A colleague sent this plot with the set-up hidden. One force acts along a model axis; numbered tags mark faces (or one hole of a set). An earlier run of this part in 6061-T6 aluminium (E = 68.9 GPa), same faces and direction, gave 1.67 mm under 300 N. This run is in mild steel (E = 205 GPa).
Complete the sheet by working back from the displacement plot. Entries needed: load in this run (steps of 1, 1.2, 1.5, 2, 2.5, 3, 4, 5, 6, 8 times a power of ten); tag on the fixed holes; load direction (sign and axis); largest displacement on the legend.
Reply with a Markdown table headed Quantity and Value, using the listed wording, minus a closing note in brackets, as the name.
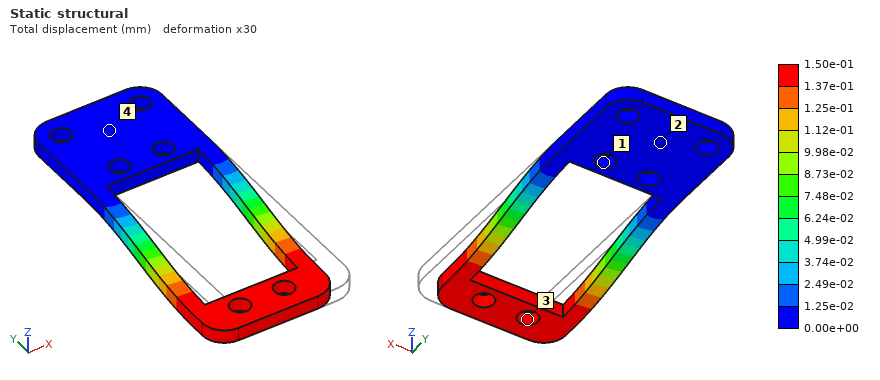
| Quantity | Value |
|---|---|
| load in this run | 80 N |
| tag on the fixed holes | 1 |
| load direction | -X |
| largest displacement on the legend | 1.50e-01 mm |
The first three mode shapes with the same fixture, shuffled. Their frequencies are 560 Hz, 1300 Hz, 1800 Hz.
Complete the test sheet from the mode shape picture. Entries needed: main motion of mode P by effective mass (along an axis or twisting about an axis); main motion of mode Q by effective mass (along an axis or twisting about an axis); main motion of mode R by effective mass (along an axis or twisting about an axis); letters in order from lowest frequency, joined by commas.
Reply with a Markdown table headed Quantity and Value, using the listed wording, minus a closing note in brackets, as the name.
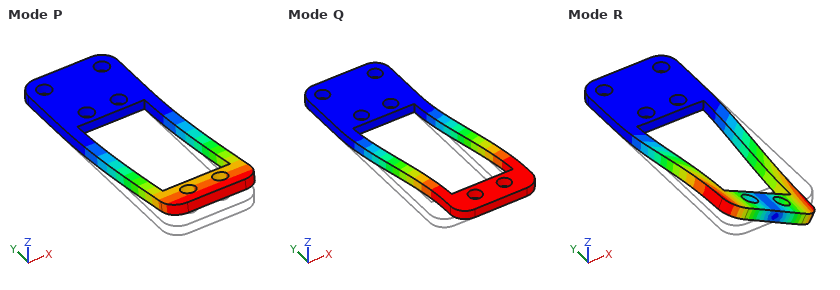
| Quantity | Value |
|---|---|
| main motion of mode P by effective mass | along Z |
| main motion of mode Q by effective mass | along X |
| main motion of mode R by effective mass | twisting about Y |
| letters in order from lowest frequency, joined by commas | P, Q, R |
